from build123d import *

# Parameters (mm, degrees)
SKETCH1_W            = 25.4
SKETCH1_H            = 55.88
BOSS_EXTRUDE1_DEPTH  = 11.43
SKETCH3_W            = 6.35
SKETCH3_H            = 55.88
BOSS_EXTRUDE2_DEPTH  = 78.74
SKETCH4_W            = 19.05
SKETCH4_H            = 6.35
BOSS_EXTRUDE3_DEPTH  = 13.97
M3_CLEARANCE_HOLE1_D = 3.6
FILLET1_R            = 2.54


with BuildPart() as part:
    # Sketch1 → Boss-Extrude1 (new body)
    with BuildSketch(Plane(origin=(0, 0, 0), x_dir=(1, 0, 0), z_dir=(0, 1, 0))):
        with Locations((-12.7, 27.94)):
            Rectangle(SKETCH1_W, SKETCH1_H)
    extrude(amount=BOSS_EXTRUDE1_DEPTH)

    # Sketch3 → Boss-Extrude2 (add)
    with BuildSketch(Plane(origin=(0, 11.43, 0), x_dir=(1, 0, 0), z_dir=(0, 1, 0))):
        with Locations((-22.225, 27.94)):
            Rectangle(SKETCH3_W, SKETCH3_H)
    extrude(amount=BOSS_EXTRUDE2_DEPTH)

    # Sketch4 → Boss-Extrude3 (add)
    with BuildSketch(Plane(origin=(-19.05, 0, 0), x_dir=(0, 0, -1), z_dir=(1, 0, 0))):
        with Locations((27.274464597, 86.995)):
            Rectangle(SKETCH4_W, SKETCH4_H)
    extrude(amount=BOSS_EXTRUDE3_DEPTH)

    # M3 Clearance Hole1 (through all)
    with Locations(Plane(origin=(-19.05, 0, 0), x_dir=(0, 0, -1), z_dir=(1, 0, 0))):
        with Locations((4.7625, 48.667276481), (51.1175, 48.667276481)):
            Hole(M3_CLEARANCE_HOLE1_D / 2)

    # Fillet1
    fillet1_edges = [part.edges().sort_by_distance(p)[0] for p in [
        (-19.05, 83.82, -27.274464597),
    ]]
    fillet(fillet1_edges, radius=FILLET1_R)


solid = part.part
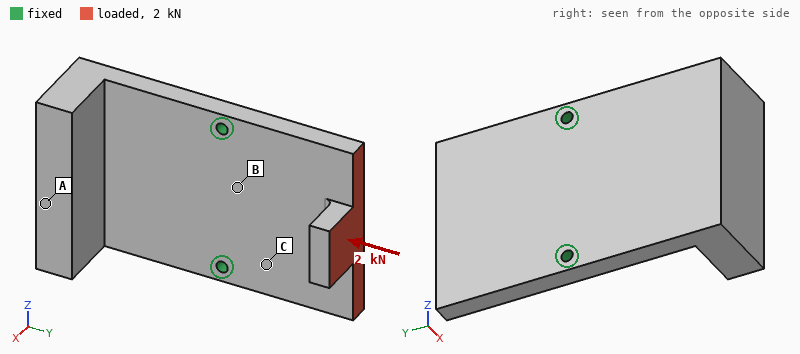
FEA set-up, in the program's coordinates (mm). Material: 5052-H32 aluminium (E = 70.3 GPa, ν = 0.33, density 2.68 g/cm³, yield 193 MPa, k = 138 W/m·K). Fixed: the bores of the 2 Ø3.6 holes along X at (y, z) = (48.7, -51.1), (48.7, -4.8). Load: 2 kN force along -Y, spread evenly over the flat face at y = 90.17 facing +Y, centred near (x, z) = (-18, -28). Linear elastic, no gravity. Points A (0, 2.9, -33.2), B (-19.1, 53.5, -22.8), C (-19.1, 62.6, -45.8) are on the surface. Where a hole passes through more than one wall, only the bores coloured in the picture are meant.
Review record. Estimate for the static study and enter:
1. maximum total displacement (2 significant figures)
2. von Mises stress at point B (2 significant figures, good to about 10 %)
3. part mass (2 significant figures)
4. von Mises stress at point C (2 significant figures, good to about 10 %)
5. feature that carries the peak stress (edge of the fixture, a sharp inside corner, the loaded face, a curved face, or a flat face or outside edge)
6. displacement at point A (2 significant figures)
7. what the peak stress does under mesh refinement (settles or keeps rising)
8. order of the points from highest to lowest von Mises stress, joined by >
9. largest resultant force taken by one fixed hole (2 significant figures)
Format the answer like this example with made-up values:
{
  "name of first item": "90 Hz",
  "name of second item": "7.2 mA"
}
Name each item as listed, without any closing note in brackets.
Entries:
{
  "maximum total displacement": "0.15 mm",
  "von Mises stress at point B": "19 MPa",
  "part mass": "120 g",
  "von Mises stress at point C": "29 MPa",
  "feature that carries the peak stress": "edge of the fixture",
  "displacement at point A": "0.030 mm",
  "what the peak stress does under mesh refinement": "keeps rising",
  "order of the points from highest to lowest von Mises stress, joined by >": "C > B > A",
  "largest resultant force taken by one fixed hole": "1.0 kN"
}
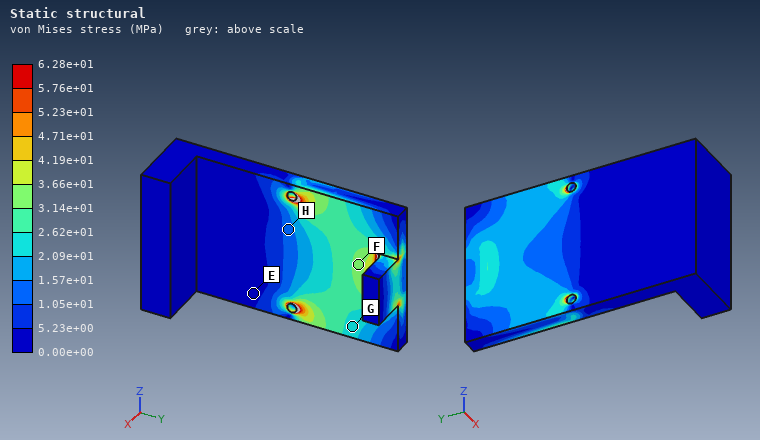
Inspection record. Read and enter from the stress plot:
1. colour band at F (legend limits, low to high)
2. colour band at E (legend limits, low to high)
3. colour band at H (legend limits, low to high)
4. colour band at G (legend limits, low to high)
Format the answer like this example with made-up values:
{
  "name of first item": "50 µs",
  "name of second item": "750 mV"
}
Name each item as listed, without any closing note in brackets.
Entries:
{
  "colour band at F": "3.14e+01 to 3.66e+01 MPa",
  "colour band at E": "0.00e+00 to 5.23e+00 MPa",
  "colour band at H": "1.05e+01 to 1.57e+01 MPa",
  "colour band at G": "2.09e+01 to 2.62e+01 MPa"
}
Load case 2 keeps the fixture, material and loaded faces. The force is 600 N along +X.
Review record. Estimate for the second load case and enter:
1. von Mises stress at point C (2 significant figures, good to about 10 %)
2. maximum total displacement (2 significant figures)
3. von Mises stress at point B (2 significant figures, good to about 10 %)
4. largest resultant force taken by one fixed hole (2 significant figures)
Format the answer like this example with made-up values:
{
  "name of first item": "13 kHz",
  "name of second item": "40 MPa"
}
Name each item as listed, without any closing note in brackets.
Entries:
{
  "von Mises stress at point C": "44 MPa",
  "maximum total displacement": "0.27 mm",
  "von Mises stress at point B": "36 MPa",
  "largest resultant force taken by one fixed hole": "300 N"
}
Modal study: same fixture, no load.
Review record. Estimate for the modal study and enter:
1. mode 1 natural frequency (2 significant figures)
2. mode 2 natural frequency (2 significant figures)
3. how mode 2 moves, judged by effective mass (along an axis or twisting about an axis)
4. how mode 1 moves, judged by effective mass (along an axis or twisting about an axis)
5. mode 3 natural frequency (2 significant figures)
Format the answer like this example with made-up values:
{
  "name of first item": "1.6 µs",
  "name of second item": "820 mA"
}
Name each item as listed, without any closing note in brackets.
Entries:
{
  "mode 1 natural frequency": "1000 Hz",
  "mode 2 natural frequency": "2200 Hz",
  "how mode 2 moves, judged by effective mass": "along X",
  "how mode 1 moves, judged by effective mass": "along X",
  "mode 3 natural frequency": "2800 Hz"
}
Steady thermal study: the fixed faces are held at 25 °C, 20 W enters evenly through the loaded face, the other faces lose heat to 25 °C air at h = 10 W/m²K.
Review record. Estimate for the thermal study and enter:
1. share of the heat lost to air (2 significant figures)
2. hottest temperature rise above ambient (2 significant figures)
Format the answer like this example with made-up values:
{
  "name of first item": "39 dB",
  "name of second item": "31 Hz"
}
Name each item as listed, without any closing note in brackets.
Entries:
{
  "share of the heat lost to air": "4.4 %",
  "hottest temperature rise above ambient": "24 K"
}
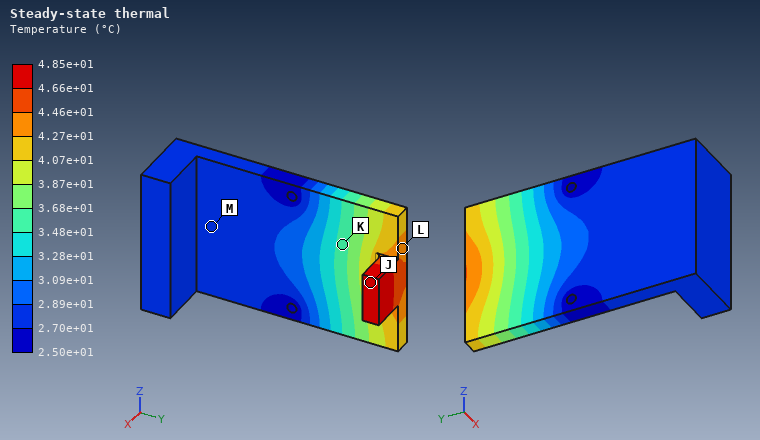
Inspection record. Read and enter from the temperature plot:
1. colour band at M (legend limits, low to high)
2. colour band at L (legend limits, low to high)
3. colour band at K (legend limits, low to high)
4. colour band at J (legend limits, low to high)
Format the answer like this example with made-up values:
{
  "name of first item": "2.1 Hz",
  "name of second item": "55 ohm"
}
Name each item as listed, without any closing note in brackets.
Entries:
{
  "colour band at M": "2.70e+01 to 2.89e+01 °C",
  "colour band at L": "4.27e+01 to 4.46e+01 °C",
  "colour band at K": "3.48e+01 to 3.68e+01 °C",
  "colour band at J": "4.66e+01 to 4.85e+01 °C"
}
